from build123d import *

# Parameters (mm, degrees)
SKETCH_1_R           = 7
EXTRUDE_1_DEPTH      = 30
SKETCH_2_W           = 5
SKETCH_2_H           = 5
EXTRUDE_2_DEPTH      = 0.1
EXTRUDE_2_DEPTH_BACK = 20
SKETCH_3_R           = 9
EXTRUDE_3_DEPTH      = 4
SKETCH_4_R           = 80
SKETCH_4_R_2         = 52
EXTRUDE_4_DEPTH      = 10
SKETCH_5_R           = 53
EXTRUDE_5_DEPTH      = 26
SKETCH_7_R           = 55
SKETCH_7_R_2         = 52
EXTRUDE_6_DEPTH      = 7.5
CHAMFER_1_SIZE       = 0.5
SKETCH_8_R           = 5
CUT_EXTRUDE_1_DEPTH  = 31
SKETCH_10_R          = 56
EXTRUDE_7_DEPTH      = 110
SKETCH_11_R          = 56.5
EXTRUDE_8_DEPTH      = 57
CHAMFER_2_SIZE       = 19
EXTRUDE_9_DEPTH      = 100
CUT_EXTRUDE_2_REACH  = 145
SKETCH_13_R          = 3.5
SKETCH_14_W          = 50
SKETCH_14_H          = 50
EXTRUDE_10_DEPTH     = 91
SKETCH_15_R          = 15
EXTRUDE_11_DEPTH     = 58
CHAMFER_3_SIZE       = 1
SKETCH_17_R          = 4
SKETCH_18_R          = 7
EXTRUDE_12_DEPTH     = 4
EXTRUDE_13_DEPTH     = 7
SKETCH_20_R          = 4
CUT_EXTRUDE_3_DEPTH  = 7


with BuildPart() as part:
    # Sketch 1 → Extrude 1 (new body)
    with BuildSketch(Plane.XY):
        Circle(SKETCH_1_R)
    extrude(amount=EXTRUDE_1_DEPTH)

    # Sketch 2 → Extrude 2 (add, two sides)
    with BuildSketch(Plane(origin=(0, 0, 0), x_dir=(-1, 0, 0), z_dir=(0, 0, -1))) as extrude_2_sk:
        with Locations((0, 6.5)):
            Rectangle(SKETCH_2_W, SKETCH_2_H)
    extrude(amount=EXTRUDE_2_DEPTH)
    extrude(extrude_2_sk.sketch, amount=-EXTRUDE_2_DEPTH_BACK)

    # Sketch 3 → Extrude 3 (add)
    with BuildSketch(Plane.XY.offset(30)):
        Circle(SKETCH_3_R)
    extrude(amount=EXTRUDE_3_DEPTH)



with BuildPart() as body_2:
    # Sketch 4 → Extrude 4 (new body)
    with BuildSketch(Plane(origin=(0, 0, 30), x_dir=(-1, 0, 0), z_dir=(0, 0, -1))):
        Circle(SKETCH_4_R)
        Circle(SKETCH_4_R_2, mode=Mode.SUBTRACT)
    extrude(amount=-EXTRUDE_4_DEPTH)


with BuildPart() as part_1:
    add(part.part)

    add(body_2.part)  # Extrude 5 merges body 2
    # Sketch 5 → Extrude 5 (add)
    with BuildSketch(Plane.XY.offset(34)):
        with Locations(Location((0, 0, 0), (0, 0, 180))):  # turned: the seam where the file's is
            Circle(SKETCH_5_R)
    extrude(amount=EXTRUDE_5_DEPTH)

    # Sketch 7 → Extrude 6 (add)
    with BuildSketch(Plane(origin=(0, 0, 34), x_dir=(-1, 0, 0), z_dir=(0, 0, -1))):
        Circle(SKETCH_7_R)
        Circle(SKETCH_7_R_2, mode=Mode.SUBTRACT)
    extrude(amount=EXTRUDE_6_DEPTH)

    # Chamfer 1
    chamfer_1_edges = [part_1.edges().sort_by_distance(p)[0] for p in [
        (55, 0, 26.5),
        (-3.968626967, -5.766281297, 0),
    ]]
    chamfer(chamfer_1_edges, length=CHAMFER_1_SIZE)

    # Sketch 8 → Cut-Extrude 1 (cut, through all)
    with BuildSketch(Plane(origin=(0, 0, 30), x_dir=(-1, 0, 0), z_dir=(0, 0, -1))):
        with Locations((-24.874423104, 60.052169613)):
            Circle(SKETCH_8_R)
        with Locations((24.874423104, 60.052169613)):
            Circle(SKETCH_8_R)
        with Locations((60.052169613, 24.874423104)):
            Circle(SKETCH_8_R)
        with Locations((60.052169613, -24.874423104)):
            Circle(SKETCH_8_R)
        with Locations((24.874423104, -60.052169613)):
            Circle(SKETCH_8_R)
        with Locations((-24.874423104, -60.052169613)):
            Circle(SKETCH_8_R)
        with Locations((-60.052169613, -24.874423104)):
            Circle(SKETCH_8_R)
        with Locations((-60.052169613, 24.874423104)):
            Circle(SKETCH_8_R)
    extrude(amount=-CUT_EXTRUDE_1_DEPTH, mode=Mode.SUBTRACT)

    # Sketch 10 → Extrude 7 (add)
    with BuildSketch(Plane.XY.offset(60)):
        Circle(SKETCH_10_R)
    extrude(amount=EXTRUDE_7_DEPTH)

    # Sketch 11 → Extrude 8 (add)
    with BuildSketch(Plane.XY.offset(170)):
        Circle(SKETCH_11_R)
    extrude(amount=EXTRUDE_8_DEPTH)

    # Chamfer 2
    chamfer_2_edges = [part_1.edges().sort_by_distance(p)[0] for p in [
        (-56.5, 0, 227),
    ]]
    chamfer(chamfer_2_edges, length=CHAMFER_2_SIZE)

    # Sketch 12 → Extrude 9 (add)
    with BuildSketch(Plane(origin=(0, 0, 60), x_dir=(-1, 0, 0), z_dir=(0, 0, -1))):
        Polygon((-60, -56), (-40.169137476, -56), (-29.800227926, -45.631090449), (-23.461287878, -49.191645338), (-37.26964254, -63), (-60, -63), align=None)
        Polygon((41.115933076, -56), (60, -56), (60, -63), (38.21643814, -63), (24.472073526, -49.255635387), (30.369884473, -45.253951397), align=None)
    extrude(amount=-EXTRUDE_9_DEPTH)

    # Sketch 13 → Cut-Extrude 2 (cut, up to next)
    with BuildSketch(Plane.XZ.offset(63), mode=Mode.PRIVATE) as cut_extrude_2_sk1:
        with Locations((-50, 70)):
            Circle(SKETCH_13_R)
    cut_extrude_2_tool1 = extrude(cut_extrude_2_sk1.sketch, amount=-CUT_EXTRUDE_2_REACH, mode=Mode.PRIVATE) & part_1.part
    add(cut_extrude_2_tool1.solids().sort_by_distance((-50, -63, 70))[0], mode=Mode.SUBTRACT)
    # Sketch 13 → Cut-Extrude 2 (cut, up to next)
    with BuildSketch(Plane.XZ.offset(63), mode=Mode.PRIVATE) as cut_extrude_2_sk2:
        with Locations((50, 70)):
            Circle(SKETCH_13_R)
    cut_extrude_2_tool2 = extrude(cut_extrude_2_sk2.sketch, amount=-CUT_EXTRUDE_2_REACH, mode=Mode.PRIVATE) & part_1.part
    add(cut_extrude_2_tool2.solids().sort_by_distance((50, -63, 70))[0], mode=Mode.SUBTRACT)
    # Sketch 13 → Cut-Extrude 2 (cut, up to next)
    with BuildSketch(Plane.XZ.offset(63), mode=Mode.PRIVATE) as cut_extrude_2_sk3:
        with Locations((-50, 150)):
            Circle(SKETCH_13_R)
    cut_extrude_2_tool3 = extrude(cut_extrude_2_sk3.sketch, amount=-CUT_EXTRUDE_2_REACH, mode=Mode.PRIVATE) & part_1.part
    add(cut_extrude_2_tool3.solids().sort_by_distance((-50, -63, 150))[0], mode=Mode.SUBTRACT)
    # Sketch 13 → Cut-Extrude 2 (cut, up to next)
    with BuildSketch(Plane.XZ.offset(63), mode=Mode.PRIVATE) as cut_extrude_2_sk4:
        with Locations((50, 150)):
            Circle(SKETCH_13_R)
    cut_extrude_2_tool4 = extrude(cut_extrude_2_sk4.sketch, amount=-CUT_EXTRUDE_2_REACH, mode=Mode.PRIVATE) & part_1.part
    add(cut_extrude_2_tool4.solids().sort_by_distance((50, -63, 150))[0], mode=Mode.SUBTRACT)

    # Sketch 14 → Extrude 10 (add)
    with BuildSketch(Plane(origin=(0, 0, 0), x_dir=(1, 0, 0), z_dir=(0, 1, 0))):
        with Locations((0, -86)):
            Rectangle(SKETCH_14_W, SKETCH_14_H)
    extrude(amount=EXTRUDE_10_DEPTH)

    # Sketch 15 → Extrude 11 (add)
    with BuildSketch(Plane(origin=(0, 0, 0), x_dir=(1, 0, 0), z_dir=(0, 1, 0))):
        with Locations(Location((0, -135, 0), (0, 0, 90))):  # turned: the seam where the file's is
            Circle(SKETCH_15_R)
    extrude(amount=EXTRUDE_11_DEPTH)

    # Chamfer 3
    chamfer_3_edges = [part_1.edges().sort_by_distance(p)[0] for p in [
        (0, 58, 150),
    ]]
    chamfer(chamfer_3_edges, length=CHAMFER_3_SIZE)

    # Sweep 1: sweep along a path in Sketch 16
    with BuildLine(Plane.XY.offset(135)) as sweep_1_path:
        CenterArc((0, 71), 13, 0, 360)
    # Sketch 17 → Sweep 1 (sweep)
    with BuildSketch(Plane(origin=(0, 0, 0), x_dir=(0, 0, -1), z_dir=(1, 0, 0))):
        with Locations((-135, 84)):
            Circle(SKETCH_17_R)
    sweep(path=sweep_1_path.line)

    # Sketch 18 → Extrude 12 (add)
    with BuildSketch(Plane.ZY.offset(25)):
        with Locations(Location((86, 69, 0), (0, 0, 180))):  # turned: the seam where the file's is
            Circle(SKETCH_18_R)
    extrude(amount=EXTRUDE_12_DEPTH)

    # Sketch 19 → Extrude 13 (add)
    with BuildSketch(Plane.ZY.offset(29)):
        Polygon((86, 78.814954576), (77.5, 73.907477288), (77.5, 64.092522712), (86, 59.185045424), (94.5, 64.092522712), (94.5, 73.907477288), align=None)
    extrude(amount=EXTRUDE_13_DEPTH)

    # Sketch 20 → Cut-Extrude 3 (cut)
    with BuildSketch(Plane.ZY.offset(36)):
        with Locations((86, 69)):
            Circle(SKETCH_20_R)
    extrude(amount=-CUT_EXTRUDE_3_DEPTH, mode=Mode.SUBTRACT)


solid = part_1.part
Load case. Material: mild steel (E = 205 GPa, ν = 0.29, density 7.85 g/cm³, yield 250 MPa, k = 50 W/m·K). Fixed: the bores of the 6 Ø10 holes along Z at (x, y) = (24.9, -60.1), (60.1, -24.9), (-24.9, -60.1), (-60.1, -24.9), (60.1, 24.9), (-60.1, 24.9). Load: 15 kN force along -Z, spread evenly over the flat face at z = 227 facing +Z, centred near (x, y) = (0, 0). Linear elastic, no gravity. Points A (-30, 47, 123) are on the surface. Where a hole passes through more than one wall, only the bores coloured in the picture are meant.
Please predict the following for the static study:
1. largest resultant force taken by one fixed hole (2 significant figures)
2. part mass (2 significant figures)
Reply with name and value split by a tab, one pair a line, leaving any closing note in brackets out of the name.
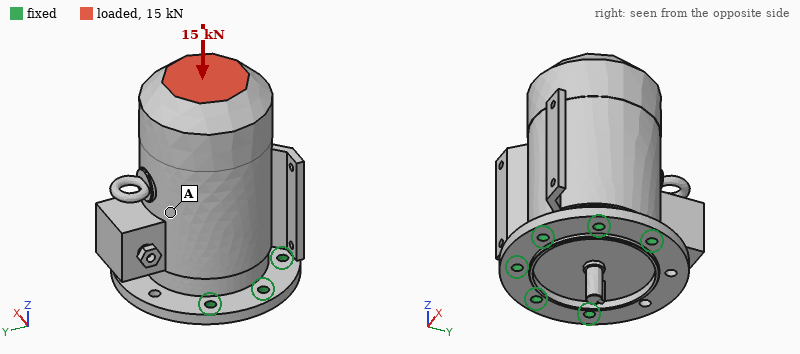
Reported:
largest resultant force taken by one fixed hole	4.9 kN
part mass	16 kg
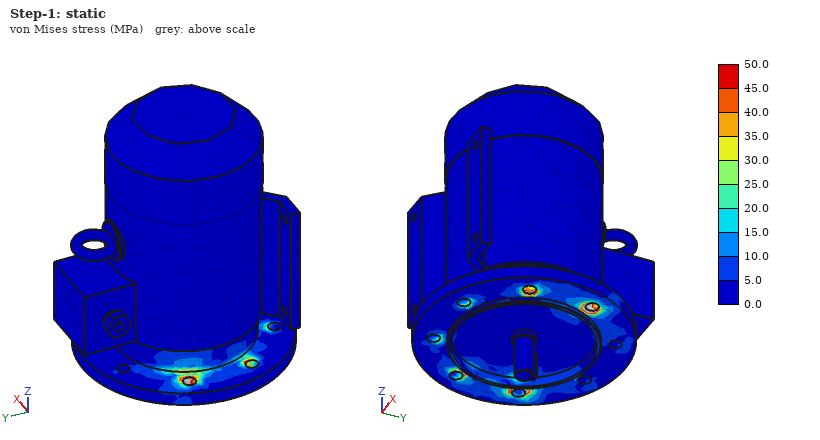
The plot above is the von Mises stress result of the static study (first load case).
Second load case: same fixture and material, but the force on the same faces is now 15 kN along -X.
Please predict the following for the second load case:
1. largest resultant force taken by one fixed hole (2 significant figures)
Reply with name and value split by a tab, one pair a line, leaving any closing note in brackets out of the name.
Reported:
largest resultant force taken by one fixed hole	14 kN
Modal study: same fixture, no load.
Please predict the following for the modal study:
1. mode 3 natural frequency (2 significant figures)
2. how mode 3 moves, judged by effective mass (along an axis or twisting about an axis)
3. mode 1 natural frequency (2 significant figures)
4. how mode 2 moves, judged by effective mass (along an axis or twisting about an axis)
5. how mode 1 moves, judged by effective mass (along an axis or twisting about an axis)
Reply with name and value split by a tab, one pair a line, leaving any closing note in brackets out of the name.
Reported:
mode 3 natural frequency	2500 Hz
how mode 3 moves, judged by effective mass	along Z
mode 1 natural frequency	690 Hz
how mode 2 moves, judged by effective mass	along X
how mode 1 moves, judged by effective mass	along Y
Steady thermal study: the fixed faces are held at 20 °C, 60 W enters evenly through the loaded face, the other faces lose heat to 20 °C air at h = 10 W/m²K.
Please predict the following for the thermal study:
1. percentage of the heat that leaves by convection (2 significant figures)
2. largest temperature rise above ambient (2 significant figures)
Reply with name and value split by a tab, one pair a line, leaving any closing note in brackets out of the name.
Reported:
percentage of the heat that leaves by convection	30 %
largest temperature rise above ambient	31 K
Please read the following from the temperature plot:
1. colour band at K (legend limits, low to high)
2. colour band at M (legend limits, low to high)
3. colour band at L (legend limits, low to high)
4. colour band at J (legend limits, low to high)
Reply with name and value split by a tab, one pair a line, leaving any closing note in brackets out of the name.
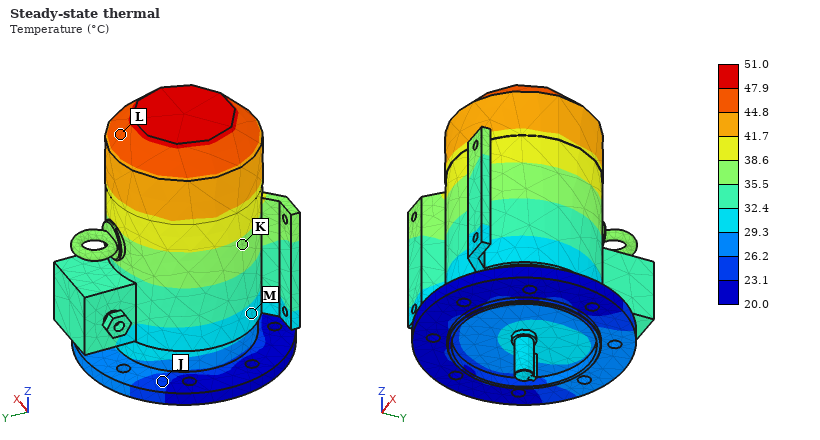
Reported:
colour band at K	35.5 to 38.6 °C
colour band at M	29.3 to 32.4 °C
colour band at L	44.8 to 47.9 °C
colour band at J	23.1 to 26.2 °C
